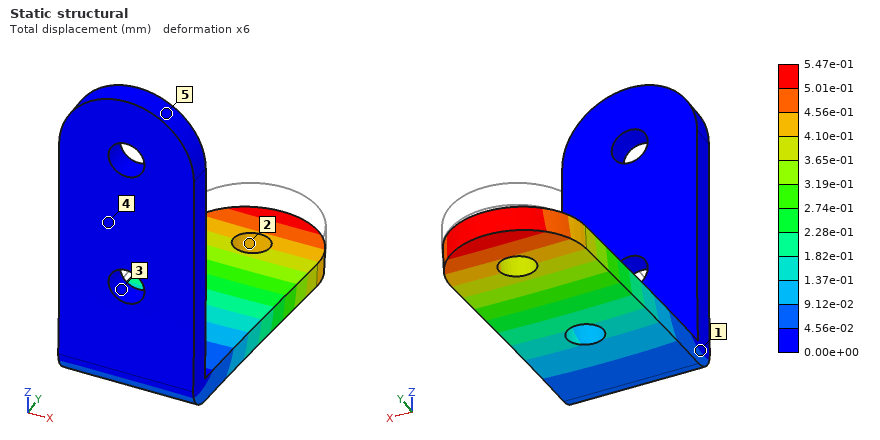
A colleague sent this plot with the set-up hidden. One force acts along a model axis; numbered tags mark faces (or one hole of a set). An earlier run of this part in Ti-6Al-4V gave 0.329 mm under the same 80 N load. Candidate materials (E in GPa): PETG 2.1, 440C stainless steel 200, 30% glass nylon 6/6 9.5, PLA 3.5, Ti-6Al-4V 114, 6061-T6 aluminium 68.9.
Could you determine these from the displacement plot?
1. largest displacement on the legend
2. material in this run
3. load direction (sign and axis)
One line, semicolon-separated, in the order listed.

5.47e-01 mm; 6061-T6 aluminium; -Z
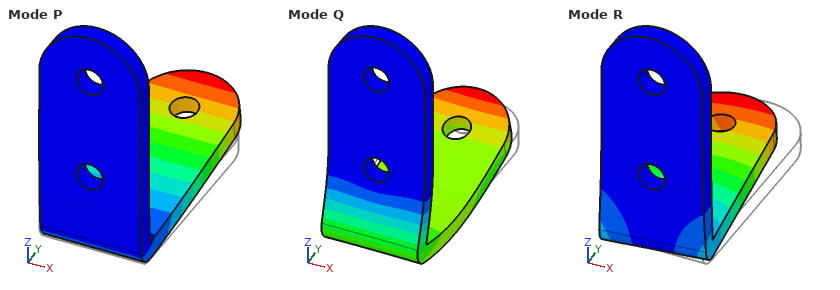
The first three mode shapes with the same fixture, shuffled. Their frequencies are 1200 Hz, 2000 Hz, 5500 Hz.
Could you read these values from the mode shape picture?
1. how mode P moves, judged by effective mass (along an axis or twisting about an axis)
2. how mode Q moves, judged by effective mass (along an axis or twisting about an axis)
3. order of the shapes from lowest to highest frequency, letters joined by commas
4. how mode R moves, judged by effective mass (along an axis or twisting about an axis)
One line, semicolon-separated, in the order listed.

along Z; along Y; P, R, Q; along X
